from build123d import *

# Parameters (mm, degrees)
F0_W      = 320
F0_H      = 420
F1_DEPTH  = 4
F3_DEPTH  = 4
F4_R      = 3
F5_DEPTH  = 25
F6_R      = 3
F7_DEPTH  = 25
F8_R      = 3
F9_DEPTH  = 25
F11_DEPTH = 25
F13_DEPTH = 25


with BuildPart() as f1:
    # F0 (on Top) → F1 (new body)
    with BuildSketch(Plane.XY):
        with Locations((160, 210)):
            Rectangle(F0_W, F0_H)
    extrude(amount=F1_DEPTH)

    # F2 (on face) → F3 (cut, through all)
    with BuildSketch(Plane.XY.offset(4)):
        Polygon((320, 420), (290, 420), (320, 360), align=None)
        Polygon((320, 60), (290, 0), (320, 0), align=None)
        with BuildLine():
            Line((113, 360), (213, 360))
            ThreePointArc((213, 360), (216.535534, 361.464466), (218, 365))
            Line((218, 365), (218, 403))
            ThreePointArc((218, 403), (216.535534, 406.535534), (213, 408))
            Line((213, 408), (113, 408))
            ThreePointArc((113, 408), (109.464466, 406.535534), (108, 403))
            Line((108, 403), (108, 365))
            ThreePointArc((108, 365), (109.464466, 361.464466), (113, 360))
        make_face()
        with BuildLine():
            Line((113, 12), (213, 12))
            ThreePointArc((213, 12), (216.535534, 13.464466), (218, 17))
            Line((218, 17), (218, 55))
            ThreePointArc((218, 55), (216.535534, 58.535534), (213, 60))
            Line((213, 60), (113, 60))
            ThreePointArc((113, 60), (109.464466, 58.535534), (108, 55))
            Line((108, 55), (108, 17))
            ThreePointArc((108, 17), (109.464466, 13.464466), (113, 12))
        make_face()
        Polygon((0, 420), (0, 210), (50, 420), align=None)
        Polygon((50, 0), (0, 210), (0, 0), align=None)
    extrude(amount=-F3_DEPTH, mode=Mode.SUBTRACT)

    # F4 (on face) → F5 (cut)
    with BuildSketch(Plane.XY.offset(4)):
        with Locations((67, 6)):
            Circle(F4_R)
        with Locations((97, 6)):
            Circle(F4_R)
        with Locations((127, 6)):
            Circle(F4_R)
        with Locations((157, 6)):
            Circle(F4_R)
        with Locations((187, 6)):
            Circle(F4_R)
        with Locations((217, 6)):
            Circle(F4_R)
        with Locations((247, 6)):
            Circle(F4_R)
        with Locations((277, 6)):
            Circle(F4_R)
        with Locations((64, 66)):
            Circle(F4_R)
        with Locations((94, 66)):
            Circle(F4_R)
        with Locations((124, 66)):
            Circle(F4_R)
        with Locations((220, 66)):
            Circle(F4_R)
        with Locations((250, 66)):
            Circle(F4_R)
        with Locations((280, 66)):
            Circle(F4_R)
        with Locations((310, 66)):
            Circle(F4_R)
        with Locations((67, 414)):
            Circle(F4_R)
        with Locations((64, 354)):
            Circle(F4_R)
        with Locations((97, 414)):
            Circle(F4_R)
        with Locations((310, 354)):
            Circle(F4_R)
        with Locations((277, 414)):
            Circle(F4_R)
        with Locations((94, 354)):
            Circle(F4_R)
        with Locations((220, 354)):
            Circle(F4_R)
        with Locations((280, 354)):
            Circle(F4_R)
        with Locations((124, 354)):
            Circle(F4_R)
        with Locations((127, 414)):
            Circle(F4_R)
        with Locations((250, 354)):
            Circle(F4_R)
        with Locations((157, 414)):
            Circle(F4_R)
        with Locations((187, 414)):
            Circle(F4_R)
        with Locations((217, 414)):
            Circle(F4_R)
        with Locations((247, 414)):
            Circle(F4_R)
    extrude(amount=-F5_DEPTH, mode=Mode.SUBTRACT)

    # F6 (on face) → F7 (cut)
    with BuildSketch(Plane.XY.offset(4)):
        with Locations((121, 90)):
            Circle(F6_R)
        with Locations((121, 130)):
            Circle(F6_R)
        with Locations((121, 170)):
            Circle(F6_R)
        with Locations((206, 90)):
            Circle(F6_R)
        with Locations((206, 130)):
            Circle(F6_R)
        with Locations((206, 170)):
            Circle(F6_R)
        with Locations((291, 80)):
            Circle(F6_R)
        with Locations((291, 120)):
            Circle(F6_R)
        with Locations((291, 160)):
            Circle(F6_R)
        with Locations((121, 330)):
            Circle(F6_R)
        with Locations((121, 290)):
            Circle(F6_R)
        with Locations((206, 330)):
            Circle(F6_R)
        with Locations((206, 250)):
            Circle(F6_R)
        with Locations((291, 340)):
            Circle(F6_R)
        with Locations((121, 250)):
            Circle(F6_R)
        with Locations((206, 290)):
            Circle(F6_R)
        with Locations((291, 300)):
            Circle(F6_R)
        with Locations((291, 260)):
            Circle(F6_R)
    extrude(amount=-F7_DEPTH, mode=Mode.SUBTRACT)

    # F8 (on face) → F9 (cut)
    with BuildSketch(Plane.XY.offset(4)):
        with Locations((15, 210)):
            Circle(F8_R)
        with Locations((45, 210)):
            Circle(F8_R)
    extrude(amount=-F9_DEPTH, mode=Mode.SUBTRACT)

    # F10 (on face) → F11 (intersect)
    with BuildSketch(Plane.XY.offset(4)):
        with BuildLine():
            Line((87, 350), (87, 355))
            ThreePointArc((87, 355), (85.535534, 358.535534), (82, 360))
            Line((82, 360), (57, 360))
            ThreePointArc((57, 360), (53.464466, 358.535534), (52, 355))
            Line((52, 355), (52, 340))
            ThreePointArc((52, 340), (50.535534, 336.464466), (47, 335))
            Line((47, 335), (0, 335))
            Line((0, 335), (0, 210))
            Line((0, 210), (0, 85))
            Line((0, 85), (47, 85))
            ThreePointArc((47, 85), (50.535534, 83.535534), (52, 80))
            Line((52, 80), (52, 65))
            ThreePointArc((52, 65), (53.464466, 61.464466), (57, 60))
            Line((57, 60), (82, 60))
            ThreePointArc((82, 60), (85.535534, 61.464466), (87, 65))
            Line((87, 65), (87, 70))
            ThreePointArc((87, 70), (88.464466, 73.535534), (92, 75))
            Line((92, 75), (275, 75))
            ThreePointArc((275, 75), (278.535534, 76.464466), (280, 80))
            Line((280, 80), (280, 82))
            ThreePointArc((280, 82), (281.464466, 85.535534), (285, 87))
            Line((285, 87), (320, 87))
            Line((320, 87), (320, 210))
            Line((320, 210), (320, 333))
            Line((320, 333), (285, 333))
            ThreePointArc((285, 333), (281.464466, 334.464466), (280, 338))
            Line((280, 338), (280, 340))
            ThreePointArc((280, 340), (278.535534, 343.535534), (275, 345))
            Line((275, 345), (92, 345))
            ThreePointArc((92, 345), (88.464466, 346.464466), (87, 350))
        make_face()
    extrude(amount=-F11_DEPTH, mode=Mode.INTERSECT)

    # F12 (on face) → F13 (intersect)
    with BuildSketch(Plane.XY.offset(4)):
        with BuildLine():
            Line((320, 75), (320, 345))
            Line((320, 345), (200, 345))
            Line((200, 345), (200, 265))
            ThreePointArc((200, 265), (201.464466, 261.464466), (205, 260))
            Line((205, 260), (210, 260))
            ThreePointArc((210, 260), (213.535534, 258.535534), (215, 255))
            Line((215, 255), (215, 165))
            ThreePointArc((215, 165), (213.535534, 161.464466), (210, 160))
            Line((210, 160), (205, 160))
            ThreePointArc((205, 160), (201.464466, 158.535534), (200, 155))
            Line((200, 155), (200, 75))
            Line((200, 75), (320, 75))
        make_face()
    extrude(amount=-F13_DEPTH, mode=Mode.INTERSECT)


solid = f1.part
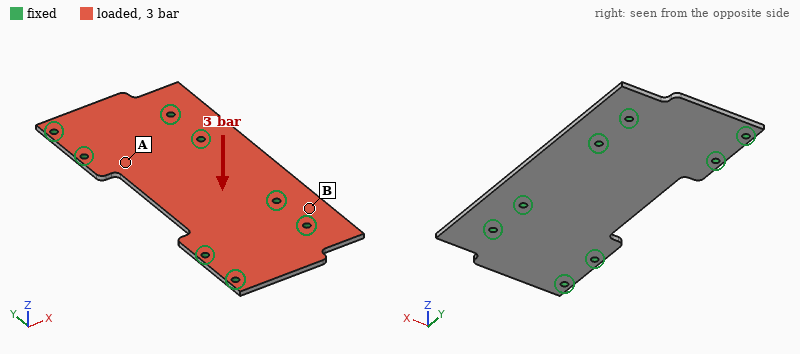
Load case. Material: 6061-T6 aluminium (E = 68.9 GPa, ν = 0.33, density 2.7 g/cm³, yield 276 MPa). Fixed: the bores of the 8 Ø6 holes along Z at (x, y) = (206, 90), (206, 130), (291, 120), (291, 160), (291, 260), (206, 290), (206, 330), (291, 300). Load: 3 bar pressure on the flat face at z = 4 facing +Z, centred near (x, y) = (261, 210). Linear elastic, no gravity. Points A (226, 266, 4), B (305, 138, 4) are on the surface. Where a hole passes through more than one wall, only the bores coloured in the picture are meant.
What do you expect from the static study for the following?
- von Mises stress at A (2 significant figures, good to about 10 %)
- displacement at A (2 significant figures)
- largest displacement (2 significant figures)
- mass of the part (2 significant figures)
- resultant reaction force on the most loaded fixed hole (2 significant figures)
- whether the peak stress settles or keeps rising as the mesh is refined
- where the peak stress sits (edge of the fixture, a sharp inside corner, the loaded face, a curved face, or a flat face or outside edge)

67 MPa
0.33 mm
1.1 mm
320 g
1.8 kN
keeps rising
edge of the fixture
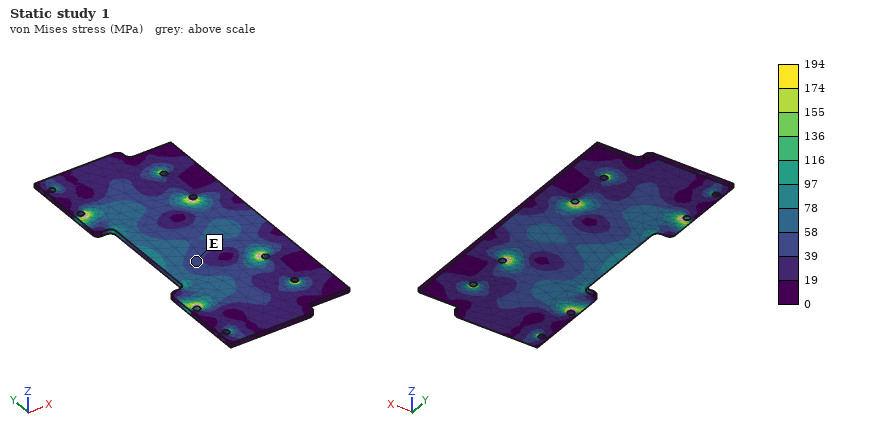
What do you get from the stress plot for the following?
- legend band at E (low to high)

39 to 58 MPa
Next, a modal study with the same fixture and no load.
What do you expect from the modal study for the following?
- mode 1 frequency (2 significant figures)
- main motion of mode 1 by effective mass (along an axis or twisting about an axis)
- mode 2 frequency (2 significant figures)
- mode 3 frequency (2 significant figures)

1100 Hz
along Z
1900 Hz
2000 Hz
